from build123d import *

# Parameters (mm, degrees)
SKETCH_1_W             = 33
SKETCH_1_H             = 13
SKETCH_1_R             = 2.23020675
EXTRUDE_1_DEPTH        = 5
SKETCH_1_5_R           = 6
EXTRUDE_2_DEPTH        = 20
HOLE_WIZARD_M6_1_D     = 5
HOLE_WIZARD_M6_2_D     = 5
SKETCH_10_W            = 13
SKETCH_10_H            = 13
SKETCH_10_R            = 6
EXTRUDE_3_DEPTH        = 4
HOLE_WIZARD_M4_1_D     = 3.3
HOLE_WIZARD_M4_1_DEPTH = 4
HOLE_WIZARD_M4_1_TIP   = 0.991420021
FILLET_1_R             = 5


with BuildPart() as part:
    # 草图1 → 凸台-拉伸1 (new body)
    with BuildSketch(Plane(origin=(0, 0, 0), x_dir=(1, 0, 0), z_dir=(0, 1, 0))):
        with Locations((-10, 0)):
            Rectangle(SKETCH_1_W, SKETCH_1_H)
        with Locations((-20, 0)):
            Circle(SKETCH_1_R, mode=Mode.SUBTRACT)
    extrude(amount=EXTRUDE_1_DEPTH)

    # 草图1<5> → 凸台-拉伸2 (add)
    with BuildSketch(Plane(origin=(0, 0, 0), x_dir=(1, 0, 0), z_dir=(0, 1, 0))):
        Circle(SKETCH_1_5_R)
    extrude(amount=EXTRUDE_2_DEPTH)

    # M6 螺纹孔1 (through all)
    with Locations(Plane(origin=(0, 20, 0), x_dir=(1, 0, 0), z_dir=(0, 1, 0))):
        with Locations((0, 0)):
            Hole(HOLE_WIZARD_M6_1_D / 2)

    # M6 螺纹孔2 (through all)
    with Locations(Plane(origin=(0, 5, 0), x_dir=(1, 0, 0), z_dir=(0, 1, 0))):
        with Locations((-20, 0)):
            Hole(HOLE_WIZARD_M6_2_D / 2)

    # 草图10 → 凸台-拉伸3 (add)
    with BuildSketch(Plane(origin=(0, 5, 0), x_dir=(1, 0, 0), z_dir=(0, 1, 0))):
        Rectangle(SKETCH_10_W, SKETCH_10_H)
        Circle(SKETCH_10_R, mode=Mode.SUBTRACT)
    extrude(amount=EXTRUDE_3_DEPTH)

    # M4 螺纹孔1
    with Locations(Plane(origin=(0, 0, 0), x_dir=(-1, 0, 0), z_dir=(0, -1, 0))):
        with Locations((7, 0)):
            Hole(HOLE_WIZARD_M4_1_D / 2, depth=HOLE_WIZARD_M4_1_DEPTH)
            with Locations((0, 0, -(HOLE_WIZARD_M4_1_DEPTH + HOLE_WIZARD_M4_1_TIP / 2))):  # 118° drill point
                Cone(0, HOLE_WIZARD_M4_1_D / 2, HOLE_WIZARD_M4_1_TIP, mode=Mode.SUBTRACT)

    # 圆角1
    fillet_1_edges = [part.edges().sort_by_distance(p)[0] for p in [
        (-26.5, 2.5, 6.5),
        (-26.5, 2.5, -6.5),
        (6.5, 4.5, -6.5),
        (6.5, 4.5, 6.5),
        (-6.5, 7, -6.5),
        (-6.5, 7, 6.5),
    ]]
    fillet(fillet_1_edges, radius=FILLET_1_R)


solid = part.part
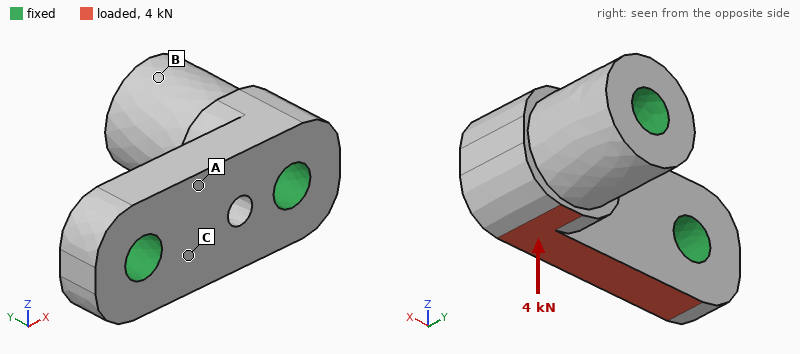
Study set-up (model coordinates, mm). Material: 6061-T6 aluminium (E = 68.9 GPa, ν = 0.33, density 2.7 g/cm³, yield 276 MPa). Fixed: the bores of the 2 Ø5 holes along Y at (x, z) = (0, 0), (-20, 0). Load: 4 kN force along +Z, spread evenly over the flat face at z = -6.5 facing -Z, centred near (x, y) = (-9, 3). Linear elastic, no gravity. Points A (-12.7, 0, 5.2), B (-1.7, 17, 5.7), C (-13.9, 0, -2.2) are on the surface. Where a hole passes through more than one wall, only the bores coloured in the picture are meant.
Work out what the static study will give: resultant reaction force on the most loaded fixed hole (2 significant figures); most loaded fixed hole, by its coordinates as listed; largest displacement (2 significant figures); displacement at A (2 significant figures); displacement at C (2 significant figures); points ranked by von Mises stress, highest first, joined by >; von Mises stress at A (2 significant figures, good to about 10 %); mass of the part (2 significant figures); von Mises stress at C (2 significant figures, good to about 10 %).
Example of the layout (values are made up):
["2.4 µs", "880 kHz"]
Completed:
["2.3 kN", "(0, 0)", "7.9 µm", "4.1 µm", "4.7 µm", "C > A > B", "16 MPa", "9.0 g", "31 MPa"]
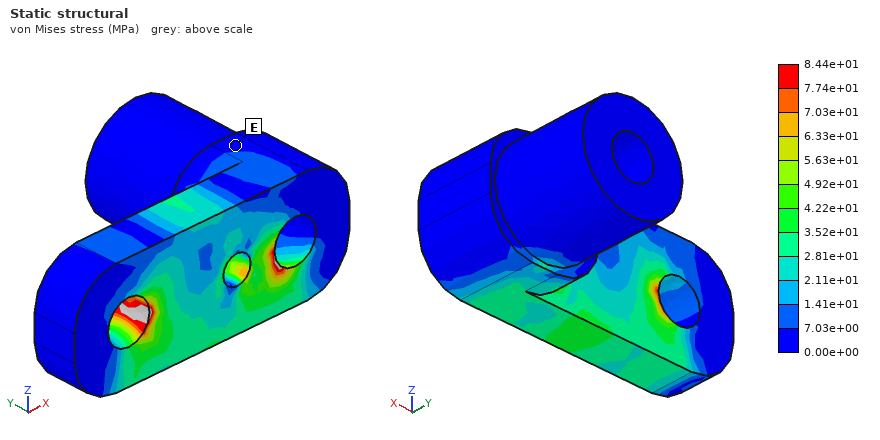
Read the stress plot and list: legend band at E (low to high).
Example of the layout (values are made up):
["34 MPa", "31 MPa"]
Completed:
["0.00e+00 to 7.03e+00 MPa"]
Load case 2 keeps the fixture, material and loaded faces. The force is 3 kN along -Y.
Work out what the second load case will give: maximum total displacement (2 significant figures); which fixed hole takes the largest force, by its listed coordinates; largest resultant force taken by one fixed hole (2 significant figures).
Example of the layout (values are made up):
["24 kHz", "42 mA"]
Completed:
["24 µm", "(0, 0)", "1.8 kN"]
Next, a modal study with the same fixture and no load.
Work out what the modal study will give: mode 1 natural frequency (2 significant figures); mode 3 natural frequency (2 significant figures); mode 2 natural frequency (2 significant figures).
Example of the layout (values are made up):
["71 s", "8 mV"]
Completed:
["67 kHz", "76 kHz", "69 kHz"]
